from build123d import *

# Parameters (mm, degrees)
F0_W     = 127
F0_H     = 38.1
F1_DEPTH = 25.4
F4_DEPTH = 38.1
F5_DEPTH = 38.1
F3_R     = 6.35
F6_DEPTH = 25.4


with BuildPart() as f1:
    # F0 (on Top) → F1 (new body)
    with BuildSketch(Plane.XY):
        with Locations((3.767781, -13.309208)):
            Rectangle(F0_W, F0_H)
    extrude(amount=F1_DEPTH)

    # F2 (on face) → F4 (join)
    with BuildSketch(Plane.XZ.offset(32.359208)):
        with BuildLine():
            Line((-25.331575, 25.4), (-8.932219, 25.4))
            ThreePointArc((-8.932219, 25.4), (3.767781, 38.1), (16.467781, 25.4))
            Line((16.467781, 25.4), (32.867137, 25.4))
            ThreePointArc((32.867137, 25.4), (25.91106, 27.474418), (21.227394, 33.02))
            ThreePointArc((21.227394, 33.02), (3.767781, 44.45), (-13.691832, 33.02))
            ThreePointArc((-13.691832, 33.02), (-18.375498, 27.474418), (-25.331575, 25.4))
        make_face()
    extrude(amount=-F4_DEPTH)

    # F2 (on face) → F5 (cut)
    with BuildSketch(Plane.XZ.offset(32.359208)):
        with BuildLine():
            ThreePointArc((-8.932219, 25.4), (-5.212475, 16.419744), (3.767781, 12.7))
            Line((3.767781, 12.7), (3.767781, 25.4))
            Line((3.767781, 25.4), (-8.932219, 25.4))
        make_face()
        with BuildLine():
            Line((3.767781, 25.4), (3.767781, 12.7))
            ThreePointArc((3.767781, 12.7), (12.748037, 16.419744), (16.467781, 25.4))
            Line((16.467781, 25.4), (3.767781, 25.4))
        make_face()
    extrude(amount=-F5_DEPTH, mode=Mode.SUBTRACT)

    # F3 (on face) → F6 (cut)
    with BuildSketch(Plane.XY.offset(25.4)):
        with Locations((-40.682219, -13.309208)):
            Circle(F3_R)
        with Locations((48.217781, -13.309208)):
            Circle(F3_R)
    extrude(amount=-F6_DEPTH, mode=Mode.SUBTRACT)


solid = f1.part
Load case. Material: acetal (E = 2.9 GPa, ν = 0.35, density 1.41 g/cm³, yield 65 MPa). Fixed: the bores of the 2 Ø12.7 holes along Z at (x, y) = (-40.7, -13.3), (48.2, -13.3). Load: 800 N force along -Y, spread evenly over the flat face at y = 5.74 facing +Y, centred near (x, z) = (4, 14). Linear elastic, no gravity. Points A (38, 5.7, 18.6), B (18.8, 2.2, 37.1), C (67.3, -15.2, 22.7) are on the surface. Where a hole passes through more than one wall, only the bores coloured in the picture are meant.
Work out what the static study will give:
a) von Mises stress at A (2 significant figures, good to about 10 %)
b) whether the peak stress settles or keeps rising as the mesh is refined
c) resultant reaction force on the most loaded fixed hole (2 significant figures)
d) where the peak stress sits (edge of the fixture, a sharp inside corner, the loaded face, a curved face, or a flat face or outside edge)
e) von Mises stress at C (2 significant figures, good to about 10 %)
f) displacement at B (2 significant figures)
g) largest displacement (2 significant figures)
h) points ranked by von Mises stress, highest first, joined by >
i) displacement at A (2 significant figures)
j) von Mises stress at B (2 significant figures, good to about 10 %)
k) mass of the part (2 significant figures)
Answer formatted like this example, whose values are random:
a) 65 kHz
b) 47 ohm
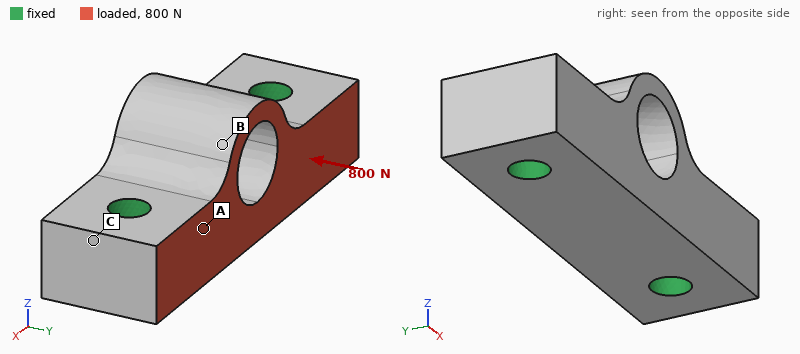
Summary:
a) 0.51 MPa
b) keeps rising
c) 400 N
d) edge of the fixture
e) 0.16 MPa
f) 17 µm
g) 23 µm
h) A > B > C
i) 6.7 µm
j) 0.34 MPa
k) 170 g
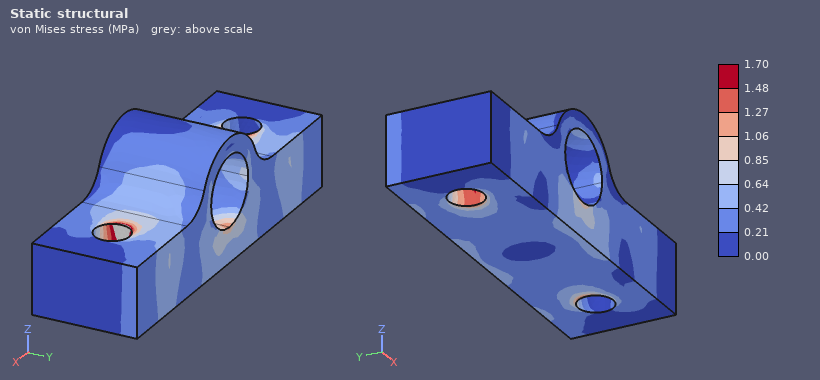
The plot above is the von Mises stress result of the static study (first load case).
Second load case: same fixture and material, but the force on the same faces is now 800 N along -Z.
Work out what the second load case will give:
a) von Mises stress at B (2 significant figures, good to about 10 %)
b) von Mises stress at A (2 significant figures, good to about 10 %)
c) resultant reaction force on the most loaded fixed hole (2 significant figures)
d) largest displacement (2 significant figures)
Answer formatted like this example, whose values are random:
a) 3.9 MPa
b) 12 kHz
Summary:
a) 0.65 MPa
b) 1.2 MPa
c) 400 N
d) 42 µm
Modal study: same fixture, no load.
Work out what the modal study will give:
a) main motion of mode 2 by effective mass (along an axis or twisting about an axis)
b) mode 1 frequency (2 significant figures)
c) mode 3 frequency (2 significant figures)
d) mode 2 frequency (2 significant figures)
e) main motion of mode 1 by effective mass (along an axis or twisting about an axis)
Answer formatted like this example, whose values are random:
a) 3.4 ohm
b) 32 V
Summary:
a) along Z
b) 2900 Hz
c) 3700 Hz
d) 3400 Hz
e) along Y
